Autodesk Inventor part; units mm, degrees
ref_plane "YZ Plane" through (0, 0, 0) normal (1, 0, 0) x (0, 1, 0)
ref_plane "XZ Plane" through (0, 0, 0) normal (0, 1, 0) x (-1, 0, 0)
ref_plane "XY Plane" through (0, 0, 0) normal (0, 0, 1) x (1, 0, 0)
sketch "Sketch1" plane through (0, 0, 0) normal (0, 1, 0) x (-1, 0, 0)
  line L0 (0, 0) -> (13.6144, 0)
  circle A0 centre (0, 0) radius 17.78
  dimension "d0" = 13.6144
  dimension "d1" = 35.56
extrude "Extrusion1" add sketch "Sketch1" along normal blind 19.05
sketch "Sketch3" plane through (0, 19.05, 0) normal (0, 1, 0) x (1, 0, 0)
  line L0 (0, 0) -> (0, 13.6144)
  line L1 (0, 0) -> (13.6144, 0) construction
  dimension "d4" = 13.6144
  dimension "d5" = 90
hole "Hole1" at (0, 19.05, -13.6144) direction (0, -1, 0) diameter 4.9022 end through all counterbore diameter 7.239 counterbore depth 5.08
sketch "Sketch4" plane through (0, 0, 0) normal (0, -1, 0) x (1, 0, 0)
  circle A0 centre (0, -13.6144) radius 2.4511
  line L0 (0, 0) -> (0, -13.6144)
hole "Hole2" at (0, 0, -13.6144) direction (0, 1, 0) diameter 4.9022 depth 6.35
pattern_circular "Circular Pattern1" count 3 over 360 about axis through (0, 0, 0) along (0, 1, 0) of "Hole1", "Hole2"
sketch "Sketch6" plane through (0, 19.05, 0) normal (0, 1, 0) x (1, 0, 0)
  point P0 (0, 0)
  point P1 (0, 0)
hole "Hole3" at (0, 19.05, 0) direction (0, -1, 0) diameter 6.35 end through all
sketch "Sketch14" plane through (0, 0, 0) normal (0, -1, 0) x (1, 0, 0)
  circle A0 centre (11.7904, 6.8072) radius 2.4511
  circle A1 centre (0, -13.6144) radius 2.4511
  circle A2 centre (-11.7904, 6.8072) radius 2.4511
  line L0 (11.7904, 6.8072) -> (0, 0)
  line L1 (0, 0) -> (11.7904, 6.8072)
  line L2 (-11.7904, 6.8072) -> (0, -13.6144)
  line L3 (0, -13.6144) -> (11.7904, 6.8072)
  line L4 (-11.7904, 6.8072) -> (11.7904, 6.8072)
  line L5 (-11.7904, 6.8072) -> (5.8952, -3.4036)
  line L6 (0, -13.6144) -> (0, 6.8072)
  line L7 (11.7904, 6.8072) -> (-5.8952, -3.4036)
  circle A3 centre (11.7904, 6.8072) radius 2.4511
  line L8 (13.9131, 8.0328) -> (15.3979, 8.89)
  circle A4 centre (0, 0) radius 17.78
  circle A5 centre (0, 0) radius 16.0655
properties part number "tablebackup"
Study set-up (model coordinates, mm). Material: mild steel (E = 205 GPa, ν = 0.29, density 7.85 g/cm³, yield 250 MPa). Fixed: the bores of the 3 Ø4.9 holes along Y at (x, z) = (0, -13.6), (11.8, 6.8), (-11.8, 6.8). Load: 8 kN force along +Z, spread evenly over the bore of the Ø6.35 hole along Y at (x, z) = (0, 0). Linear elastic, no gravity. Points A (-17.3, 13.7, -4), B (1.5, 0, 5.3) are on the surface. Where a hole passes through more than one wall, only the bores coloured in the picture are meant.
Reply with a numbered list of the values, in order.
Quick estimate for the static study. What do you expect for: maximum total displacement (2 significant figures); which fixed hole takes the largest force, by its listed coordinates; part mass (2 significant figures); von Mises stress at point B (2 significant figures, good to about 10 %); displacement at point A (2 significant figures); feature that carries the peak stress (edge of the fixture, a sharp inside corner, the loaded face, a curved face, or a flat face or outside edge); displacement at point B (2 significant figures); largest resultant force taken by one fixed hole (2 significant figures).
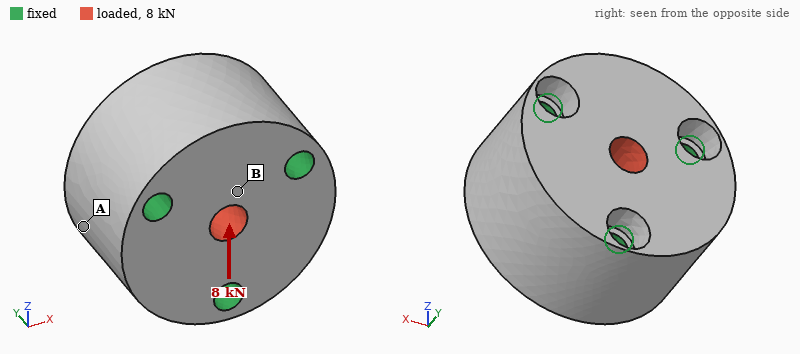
1. 1.7 µm
2. (0, -13.6)
3. 130 g
4. 17 MPa
5. 0.33 µm
6. edge of the fixture
7. 1.0 µm
8. 3.0 kN
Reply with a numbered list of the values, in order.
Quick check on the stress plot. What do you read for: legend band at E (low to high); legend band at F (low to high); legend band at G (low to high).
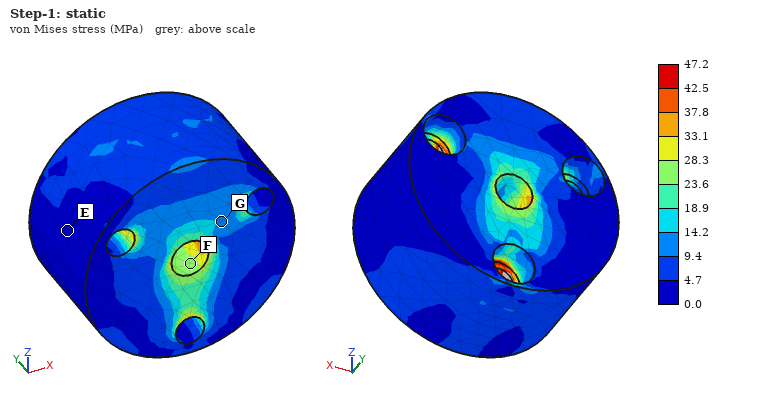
1. 0.0 to 4.7 MPa
2. 23.6 to 28.3 MPa
3. 9.4 to 14.2 MPa
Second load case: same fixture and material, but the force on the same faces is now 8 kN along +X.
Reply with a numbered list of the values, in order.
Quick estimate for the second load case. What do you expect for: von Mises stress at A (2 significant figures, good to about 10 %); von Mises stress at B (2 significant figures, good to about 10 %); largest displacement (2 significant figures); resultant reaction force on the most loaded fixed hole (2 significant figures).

1. 8.0 MPa
2. 14 MPa
3. 1.6 µm
4. 2.9 kN
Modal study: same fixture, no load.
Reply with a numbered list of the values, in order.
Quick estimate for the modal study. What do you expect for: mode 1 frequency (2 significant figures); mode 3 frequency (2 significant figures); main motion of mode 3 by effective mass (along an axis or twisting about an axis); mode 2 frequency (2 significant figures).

1. 41 kHz
2. 48 kHz
3. along Y
4. 41 kHz
